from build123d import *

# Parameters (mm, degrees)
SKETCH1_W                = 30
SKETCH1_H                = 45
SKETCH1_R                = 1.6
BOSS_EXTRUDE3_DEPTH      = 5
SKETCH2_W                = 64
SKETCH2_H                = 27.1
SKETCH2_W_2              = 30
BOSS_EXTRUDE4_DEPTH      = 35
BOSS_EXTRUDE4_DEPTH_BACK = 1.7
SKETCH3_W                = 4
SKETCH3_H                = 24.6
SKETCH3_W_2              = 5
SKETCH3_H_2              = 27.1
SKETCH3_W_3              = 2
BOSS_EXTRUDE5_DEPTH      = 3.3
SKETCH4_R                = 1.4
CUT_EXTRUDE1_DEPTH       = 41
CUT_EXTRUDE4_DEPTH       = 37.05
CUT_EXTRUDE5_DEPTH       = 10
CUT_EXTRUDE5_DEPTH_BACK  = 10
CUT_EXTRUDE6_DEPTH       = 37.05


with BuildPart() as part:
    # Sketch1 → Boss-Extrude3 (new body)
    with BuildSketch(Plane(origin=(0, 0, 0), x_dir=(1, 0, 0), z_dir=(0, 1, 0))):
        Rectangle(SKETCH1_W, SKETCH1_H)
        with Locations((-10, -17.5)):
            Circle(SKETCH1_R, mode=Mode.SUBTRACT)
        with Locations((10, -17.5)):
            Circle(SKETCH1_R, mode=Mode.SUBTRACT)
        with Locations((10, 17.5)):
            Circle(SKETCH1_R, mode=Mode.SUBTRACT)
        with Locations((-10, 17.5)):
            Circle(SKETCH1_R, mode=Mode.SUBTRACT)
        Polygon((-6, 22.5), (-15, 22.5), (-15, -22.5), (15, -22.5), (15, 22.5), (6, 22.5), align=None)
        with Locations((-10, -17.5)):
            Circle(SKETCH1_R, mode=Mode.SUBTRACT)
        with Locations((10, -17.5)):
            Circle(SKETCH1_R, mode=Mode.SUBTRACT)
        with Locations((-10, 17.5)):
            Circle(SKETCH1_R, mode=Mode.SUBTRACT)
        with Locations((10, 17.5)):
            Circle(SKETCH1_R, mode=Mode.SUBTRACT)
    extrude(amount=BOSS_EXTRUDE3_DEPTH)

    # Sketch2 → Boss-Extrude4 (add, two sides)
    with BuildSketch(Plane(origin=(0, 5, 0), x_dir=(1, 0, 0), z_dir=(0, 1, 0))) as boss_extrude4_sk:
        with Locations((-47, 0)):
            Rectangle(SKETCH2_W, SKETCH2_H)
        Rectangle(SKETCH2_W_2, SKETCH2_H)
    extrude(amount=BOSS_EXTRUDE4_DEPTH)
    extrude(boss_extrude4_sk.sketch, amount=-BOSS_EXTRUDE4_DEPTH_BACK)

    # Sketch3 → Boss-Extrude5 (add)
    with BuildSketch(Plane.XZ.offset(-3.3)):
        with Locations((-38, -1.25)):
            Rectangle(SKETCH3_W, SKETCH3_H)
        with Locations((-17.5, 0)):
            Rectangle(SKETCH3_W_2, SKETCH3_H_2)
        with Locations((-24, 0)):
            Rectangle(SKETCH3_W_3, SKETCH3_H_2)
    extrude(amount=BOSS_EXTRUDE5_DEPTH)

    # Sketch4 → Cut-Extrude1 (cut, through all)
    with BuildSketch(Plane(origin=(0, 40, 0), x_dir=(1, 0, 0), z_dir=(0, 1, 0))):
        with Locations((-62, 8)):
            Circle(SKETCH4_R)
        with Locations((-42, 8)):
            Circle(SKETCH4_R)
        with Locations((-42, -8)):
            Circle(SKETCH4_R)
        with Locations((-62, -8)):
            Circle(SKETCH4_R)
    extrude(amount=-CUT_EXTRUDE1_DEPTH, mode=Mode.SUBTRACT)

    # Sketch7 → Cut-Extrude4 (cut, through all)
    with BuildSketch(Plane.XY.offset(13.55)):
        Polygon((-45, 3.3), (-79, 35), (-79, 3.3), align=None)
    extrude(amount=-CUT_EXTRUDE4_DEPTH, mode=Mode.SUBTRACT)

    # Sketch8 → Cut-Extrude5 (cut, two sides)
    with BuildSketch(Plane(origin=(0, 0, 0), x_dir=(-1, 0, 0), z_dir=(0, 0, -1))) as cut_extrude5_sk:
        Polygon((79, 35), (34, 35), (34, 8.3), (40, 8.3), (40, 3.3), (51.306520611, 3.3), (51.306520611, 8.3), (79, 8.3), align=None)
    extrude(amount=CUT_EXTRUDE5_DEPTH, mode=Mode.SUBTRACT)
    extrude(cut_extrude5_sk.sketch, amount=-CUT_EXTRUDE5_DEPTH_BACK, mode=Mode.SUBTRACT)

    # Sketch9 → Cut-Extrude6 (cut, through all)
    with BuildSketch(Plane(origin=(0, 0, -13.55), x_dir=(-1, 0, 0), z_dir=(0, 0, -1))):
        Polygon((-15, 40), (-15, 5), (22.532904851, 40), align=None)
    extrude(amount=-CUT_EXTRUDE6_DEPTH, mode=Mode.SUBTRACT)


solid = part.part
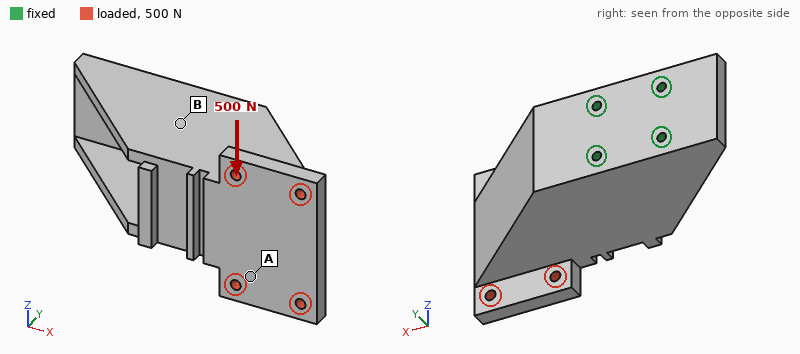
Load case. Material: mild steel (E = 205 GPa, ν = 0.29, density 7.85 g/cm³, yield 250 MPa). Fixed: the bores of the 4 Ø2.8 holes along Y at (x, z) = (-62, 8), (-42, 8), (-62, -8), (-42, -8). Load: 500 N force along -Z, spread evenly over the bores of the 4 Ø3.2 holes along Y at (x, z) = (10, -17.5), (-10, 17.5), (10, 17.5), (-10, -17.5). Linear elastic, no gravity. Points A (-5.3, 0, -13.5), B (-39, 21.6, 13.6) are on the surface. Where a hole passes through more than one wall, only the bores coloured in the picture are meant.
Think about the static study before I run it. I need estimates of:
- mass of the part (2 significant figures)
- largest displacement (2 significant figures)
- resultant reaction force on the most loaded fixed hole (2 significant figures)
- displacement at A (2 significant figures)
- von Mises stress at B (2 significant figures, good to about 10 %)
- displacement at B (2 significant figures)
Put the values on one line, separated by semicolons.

390 g; 12 µm; 990 N; 9.7 µm; 7.5 MPa; 3.6 µm
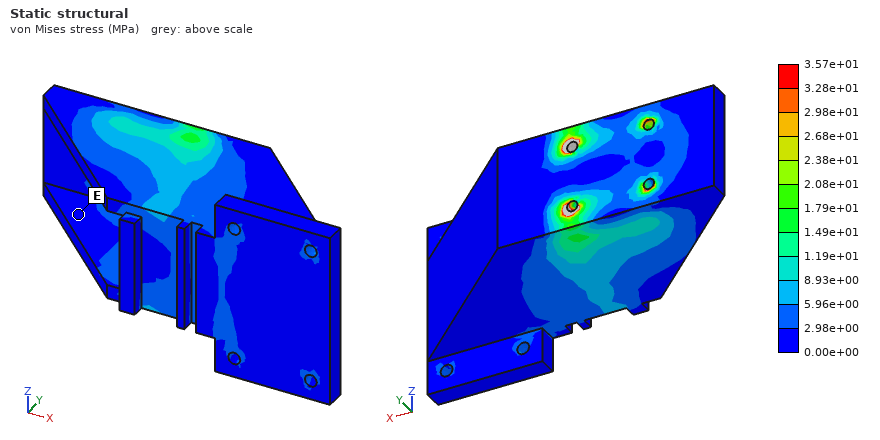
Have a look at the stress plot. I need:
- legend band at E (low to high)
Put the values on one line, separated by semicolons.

0.00e+00 to 2.98e+00 MPa
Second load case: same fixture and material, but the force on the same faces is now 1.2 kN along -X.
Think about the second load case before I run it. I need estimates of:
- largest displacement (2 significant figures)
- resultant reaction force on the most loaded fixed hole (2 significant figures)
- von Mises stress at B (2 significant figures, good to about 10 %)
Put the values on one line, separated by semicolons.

23 µm; 990 N; 12 MPa
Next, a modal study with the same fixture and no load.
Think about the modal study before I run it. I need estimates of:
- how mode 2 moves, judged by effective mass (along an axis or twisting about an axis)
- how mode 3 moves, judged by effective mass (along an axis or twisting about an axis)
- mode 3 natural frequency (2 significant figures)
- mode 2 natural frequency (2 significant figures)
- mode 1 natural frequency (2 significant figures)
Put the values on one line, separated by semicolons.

along Z; twisting about Y; 5800 Hz; 2900 Hz; 2600 Hz
